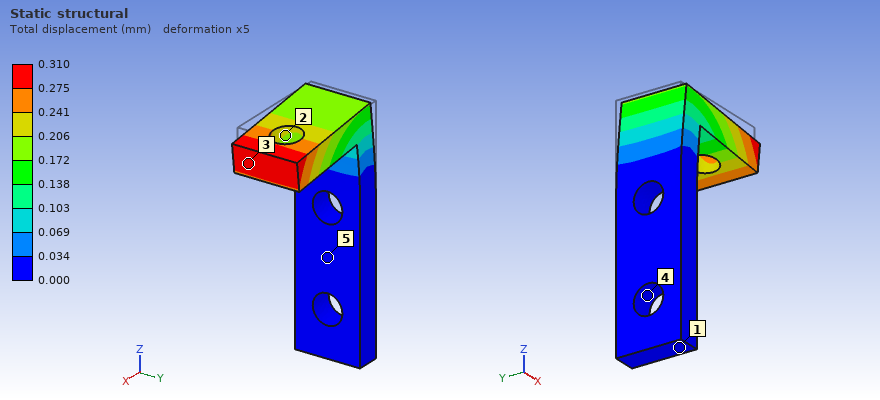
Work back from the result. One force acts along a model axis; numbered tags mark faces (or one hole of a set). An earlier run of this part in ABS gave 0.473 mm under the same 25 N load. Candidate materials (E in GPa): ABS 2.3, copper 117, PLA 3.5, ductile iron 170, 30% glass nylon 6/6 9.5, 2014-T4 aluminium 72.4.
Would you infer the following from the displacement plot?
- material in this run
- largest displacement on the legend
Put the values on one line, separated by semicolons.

PLA; 0.310 mm
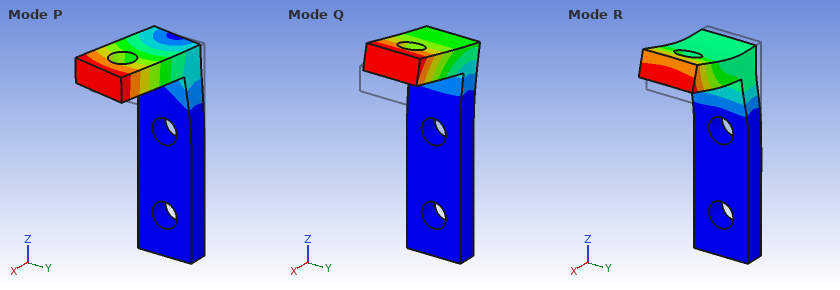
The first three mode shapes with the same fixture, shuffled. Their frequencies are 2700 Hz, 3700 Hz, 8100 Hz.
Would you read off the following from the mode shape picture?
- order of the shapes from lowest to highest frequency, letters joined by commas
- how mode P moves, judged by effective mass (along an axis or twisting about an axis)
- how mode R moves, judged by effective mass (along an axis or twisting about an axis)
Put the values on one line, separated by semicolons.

Q, P, R; along Y; along X
